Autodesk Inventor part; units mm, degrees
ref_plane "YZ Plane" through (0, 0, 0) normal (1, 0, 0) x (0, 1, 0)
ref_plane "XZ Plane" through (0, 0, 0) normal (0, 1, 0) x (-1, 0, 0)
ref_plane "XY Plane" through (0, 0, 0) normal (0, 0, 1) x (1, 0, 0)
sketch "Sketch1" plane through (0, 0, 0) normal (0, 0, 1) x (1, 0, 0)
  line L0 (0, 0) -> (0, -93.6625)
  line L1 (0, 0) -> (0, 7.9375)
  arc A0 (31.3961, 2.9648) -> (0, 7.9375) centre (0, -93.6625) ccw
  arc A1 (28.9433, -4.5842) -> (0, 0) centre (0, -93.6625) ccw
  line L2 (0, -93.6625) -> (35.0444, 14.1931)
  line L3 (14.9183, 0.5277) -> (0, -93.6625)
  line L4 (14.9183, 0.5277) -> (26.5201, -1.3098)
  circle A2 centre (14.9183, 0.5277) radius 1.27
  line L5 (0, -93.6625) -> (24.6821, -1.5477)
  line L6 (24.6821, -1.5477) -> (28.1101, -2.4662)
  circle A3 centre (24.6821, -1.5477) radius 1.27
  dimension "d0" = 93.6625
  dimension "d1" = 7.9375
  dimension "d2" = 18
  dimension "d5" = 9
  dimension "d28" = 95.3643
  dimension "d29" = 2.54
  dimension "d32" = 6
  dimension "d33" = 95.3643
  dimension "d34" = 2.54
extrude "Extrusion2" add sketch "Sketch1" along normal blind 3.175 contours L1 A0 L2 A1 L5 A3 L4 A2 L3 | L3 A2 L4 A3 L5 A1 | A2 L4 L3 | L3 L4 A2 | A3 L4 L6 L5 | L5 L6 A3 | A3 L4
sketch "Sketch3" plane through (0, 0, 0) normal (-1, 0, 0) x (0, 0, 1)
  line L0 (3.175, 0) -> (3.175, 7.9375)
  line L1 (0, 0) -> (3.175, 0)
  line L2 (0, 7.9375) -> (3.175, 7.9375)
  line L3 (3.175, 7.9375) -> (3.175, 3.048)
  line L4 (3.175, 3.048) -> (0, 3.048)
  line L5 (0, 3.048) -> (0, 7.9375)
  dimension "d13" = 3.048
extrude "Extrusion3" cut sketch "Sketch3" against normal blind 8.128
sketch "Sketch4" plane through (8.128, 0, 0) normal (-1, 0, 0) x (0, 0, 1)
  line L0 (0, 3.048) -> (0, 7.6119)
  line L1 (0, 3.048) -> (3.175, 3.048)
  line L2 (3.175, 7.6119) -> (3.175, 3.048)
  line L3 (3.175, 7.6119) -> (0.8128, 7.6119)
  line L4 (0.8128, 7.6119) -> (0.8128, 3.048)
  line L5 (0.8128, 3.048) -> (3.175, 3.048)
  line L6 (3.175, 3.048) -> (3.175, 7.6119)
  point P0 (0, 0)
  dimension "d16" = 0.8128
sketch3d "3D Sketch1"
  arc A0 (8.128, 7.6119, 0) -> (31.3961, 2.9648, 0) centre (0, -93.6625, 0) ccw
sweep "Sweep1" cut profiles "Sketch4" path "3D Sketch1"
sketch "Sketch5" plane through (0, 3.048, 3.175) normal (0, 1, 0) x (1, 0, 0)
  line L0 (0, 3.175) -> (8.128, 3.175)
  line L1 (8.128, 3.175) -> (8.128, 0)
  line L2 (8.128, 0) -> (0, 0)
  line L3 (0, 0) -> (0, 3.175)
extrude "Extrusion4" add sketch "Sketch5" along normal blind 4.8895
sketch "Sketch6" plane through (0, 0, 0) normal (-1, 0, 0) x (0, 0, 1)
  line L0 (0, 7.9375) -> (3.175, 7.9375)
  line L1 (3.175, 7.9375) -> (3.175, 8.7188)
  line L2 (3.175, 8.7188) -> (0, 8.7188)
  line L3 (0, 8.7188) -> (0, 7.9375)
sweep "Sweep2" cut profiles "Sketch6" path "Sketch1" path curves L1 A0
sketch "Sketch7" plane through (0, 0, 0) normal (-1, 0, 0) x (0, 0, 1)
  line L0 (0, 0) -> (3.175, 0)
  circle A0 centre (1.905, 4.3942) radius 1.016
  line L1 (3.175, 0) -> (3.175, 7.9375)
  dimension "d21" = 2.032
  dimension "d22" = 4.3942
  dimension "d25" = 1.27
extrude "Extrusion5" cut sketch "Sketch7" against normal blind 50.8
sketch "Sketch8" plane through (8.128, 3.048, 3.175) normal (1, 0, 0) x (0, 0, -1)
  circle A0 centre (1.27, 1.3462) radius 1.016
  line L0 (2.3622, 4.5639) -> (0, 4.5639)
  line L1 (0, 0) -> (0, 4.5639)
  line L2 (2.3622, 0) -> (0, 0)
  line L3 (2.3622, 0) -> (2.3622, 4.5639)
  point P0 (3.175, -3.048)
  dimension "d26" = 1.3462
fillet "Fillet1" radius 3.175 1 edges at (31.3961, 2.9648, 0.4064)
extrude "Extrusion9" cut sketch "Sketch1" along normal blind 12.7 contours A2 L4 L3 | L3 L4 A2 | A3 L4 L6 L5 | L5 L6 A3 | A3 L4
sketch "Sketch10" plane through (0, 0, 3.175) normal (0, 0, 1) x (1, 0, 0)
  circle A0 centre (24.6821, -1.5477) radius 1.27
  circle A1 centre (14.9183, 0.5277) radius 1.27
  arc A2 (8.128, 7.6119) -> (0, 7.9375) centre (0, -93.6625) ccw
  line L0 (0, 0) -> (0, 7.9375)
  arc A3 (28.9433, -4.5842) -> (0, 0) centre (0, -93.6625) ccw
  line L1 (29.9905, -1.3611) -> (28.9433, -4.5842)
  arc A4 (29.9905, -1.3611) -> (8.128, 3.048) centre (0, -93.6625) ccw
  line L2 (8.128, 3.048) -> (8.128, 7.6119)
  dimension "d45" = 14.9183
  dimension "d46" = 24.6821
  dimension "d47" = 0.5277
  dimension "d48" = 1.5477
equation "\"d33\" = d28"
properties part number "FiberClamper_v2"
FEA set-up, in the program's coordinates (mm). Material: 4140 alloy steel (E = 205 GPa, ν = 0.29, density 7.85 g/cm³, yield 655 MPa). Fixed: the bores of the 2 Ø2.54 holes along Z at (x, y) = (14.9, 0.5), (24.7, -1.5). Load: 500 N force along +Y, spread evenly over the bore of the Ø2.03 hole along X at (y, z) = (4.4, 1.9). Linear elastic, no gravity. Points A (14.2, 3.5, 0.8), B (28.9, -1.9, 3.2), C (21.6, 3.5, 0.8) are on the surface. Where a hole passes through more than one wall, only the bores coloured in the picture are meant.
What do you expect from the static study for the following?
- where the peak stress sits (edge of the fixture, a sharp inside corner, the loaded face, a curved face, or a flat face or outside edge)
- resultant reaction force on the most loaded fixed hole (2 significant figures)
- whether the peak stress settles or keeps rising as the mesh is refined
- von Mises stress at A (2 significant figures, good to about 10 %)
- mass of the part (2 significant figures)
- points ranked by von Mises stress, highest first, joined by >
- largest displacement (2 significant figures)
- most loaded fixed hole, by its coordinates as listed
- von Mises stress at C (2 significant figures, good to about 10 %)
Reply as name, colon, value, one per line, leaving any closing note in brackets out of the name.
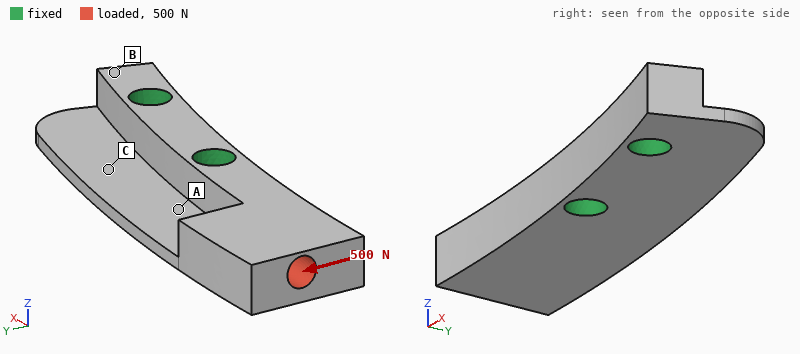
where the peak stress sits: edge of the fixture
resultant reaction force on the most loaded fixed hole: 770 N
whether the peak stress settles or keeps rising as the mesh is refined: keeps rising
von Mises stress at A: 170 MPa
mass of the part: 3.6 g
points ranked by von Mises stress, highest first, joined by >: A > C > B
largest displacement: 62 µm
most loaded fixed hole, by its coordinates as listed: (14.9, 0.5)
von Mises stress at C: 76 MPa
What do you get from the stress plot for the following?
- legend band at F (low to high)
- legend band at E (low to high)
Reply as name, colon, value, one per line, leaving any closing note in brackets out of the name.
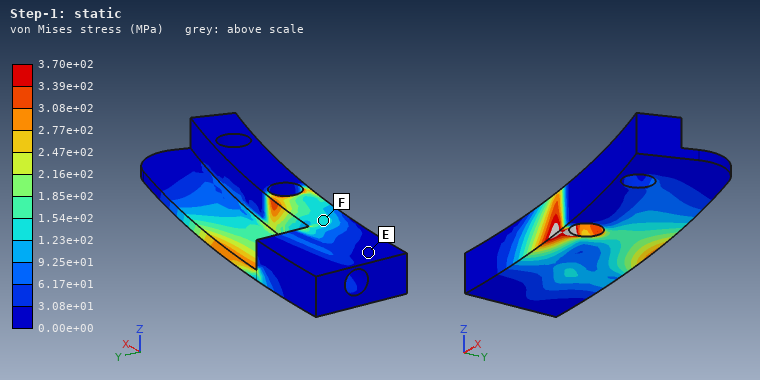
legend band at F: 1.23e+02 to 1.54e+02 MPa
legend band at E: 0.00e+00 to 3.08e+01 MPa
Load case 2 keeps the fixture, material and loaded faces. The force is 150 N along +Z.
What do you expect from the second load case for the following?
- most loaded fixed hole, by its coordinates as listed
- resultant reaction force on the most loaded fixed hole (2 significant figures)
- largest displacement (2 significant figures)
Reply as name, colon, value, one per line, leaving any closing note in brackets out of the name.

most loaded fixed hole, by its coordinates as listed: (14.9, 0.5)
resultant reaction force on the most loaded fixed hole: 150 N
largest displacement: 57 µm
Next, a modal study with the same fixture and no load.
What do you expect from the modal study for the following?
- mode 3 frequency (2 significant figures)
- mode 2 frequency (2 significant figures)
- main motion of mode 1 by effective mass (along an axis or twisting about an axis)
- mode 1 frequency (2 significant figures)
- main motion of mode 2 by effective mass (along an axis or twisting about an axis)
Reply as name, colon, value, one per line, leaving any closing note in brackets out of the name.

mode 3 frequency: 21 kHz
mode 2 frequency: 15 kHz
main motion of mode 1 by effective mass: along Z
mode 1 frequency: 8700 Hz
main motion of mode 2 by effective mass: along Y
